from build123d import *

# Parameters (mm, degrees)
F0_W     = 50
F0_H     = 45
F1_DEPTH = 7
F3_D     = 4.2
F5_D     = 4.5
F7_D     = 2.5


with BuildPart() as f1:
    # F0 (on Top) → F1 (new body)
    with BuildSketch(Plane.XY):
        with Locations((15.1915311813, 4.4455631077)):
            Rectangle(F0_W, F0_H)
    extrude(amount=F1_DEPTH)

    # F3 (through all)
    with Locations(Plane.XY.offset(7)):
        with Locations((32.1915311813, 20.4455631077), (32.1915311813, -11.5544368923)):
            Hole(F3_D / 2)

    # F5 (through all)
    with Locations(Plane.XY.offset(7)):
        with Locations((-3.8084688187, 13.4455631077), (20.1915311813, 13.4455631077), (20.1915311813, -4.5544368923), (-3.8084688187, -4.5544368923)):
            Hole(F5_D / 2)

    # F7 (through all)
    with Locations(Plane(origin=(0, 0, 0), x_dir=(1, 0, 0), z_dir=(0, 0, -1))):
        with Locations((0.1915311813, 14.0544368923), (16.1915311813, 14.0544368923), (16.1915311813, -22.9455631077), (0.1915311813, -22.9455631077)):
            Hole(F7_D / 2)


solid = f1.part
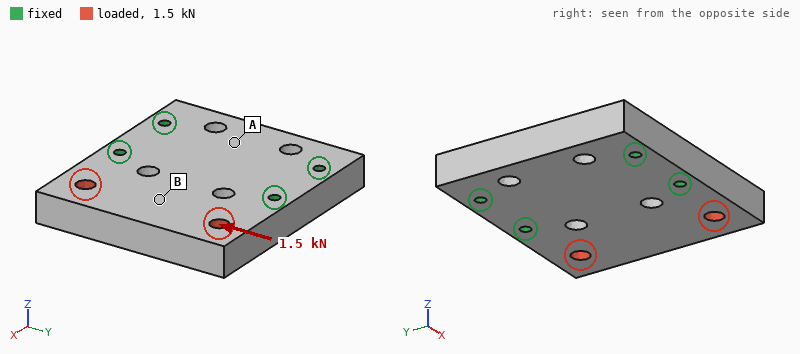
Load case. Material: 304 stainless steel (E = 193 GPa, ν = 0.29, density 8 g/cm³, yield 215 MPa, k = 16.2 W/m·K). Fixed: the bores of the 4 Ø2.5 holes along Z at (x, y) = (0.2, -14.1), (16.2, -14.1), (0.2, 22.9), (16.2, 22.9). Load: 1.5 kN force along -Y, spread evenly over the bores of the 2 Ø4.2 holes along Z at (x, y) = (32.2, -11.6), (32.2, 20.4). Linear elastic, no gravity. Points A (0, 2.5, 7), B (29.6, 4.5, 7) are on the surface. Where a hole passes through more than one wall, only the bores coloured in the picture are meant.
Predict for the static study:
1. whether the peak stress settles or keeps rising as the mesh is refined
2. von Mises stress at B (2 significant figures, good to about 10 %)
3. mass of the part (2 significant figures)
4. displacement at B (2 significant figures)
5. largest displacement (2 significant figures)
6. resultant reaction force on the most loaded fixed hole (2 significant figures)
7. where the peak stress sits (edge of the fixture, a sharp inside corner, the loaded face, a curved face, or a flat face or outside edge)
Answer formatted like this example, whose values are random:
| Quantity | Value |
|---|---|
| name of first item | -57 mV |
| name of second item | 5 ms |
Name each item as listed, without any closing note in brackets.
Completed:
| Quantity | Value |
|---|---|
| whether the peak stress settles or keeps rising as the mesh is refined | keeps rising |
| von Mises stress at B | 6.9 MPa |
| mass of the part | 120 g |
| displacement at B | 1.4 µm |
| largest displacement | 2.2 µm |
| resultant reaction force on the most loaded fixed hole | 870 N |
| where the peak stress sits | edge of the fixture |
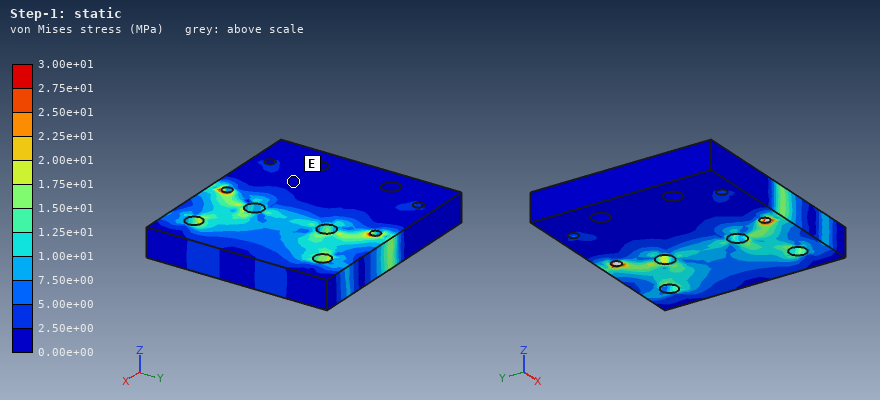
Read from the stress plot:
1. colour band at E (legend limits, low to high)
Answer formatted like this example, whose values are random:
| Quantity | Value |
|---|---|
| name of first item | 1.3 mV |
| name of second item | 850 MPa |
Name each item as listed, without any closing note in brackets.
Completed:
| Quantity | Value |
|---|---|
| colour band at E | 0.00e+00 to 2.50e+00 MPa |
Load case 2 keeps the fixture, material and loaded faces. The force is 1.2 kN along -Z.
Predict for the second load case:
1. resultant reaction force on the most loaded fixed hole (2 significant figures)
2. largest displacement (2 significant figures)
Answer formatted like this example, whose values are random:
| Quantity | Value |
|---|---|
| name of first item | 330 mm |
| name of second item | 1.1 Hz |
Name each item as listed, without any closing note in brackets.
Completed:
| Quantity | Value |
|---|---|
| resultant reaction force on the most loaded fixed hole | 820 N |
| largest displacement | 20 µm |
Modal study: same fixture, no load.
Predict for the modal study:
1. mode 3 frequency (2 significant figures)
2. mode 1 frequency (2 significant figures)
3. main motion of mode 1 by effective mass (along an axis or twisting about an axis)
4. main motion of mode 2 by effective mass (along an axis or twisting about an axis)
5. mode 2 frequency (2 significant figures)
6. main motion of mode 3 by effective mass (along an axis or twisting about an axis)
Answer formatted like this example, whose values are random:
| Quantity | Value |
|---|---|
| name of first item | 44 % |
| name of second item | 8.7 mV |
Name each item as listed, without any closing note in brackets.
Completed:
| Quantity | Value |
|---|---|
| mode 3 frequency | 18 kHz |
| mode 1 frequency | 6900 Hz |
| main motion of mode 1 by effective mass | along Z |
| main motion of mode 2 by effective mass | twisting about X |
| mode 2 frequency | 13 kHz |
| main motion of mode 3 by effective mass | along Z |
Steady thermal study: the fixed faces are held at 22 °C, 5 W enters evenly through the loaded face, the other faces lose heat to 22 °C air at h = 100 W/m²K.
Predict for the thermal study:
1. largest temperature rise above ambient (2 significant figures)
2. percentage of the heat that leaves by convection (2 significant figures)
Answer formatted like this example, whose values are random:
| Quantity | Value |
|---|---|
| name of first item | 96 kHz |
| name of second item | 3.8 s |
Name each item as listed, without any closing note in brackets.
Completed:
| Quantity | Value |
|---|---|
| largest temperature rise above ambient | 16 K |
| percentage of the heat that leaves by convection | 53 % |
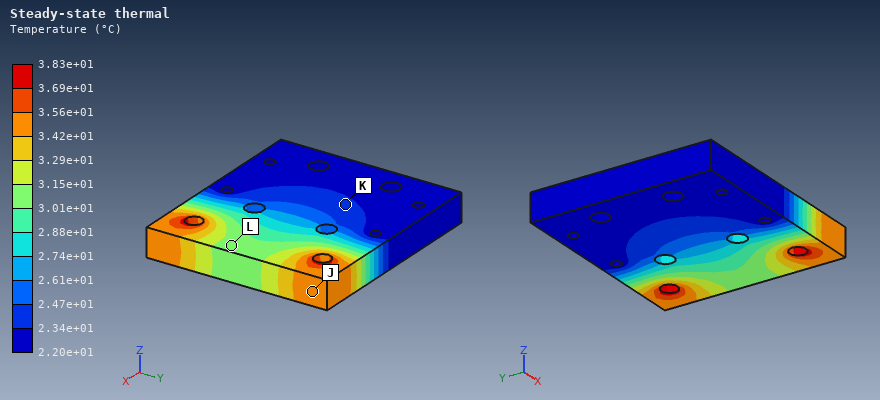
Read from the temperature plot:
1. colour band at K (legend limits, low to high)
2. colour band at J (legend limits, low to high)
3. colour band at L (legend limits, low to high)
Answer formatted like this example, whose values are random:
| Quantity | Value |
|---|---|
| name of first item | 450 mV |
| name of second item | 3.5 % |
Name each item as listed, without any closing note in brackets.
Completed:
| Quantity | Value |
|---|---|
| colour band at K | 2.34e+01 to 2.47e+01 °C |
| colour band at J | 3.42e+01 to 3.56e+01 °C |
| colour band at L | 3.01e+01 to 3.15e+01 °C |
